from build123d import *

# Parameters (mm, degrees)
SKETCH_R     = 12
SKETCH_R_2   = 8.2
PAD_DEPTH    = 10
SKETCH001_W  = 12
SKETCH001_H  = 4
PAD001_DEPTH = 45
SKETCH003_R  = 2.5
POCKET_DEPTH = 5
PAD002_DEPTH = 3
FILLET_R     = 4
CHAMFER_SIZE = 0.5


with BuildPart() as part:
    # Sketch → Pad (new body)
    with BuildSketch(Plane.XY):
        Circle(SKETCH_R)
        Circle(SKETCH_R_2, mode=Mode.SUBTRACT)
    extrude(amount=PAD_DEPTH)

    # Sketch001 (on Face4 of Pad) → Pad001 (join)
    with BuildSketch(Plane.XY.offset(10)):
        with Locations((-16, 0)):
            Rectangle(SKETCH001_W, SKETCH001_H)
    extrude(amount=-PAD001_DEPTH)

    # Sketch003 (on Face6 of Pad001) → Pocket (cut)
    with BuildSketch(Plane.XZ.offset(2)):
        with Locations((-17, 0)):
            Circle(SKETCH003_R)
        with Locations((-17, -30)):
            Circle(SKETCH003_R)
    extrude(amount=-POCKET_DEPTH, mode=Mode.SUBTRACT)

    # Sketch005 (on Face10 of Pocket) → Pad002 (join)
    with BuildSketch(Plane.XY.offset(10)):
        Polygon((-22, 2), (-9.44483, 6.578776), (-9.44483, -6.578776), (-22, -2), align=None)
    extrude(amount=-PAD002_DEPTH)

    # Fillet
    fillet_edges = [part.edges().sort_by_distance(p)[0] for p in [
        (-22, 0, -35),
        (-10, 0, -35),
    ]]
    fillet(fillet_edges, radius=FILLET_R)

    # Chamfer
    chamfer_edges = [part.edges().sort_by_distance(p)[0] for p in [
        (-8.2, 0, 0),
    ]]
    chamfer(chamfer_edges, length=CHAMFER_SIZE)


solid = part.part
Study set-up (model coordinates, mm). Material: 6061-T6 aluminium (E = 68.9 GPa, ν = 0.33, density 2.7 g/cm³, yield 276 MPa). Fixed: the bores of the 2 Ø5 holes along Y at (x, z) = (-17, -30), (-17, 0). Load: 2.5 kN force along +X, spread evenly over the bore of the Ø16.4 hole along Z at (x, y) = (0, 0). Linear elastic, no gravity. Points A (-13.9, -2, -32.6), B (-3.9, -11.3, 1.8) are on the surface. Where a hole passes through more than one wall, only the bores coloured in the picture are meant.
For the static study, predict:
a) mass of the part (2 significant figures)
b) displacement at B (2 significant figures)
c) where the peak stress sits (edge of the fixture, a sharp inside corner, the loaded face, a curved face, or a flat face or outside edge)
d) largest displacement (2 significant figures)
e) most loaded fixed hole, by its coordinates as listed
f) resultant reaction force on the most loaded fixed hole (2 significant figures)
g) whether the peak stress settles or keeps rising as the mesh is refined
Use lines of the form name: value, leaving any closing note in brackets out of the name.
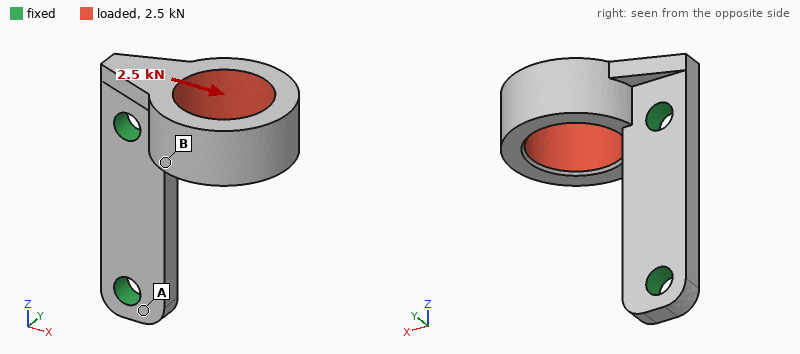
mass of the part: 12 g
displacement at B: 49 µm
where the peak stress sits: edge of the fixture
largest displacement: 80 µm
most loaded fixed hole, by its coordinates as listed: (-17, 0)
resultant reaction force on the most loaded fixed hole: 2.6 kN
whether the peak stress settles or keeps rising as the mesh is refined: keeps rising
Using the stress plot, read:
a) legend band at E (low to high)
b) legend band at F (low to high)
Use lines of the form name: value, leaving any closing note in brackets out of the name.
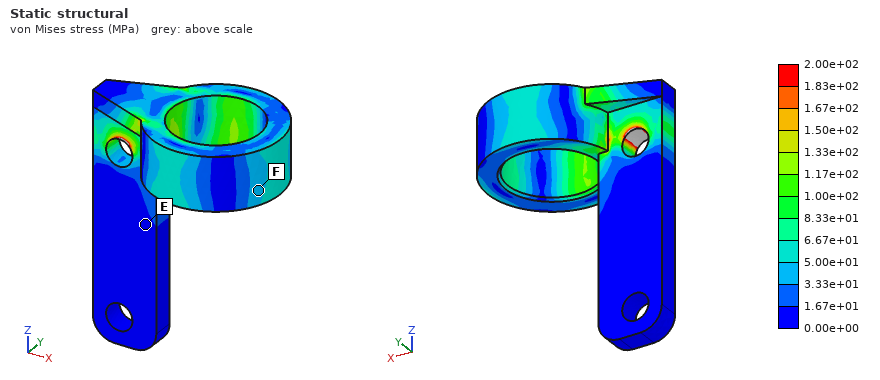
legend band at E: 0.00e+00 to 1.67e+01 MPa
legend band at F: 3.33e+01 to 5.00e+01 MPa
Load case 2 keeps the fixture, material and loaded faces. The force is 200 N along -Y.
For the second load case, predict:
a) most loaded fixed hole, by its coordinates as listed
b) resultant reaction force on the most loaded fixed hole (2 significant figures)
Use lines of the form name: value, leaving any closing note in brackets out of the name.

most loaded fixed hole, by its coordinates as listed: (-17, 0)
resultant reaction force on the most loaded fixed hole: 210 N
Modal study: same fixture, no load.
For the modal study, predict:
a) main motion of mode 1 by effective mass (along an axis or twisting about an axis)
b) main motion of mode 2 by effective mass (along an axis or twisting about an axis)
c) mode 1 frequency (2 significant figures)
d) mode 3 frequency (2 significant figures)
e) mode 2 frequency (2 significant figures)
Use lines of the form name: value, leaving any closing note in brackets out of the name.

main motion of mode 1 by effective mass: along Y
main motion of mode 2 by effective mass: along Z
mode 1 frequency: 3100 Hz
mode 3 frequency: 8800 Hz
mode 2 frequency: 5300 Hz
